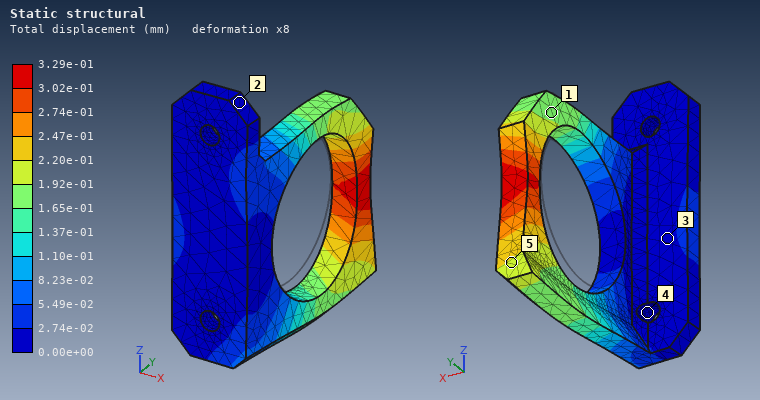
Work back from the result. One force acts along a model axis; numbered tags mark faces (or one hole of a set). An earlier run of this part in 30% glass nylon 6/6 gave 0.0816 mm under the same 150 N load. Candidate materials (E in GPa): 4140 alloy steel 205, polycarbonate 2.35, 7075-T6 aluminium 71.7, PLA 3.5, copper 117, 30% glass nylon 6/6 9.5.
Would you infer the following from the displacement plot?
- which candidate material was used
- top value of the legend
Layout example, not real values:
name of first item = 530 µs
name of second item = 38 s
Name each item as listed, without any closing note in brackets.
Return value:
which candidate material was used = polycarbonate
top value of the legend = 3.29e-01 mm
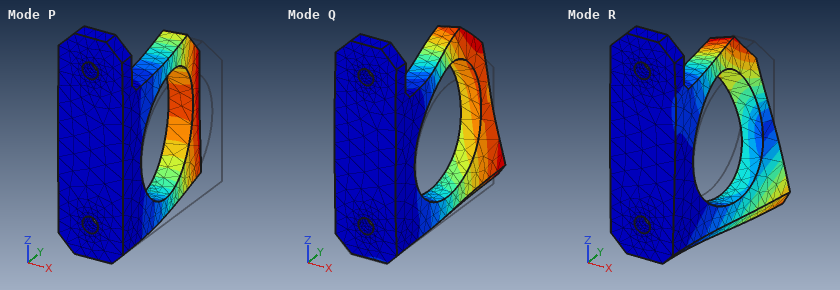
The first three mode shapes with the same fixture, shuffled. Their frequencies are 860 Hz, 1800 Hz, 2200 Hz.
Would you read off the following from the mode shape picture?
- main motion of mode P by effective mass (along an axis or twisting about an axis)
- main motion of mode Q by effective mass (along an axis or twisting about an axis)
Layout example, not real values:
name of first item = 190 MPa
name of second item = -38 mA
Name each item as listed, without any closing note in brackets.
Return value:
main motion of mode P by effective mass = along X
main motion of mode Q by effective mass = along Z
